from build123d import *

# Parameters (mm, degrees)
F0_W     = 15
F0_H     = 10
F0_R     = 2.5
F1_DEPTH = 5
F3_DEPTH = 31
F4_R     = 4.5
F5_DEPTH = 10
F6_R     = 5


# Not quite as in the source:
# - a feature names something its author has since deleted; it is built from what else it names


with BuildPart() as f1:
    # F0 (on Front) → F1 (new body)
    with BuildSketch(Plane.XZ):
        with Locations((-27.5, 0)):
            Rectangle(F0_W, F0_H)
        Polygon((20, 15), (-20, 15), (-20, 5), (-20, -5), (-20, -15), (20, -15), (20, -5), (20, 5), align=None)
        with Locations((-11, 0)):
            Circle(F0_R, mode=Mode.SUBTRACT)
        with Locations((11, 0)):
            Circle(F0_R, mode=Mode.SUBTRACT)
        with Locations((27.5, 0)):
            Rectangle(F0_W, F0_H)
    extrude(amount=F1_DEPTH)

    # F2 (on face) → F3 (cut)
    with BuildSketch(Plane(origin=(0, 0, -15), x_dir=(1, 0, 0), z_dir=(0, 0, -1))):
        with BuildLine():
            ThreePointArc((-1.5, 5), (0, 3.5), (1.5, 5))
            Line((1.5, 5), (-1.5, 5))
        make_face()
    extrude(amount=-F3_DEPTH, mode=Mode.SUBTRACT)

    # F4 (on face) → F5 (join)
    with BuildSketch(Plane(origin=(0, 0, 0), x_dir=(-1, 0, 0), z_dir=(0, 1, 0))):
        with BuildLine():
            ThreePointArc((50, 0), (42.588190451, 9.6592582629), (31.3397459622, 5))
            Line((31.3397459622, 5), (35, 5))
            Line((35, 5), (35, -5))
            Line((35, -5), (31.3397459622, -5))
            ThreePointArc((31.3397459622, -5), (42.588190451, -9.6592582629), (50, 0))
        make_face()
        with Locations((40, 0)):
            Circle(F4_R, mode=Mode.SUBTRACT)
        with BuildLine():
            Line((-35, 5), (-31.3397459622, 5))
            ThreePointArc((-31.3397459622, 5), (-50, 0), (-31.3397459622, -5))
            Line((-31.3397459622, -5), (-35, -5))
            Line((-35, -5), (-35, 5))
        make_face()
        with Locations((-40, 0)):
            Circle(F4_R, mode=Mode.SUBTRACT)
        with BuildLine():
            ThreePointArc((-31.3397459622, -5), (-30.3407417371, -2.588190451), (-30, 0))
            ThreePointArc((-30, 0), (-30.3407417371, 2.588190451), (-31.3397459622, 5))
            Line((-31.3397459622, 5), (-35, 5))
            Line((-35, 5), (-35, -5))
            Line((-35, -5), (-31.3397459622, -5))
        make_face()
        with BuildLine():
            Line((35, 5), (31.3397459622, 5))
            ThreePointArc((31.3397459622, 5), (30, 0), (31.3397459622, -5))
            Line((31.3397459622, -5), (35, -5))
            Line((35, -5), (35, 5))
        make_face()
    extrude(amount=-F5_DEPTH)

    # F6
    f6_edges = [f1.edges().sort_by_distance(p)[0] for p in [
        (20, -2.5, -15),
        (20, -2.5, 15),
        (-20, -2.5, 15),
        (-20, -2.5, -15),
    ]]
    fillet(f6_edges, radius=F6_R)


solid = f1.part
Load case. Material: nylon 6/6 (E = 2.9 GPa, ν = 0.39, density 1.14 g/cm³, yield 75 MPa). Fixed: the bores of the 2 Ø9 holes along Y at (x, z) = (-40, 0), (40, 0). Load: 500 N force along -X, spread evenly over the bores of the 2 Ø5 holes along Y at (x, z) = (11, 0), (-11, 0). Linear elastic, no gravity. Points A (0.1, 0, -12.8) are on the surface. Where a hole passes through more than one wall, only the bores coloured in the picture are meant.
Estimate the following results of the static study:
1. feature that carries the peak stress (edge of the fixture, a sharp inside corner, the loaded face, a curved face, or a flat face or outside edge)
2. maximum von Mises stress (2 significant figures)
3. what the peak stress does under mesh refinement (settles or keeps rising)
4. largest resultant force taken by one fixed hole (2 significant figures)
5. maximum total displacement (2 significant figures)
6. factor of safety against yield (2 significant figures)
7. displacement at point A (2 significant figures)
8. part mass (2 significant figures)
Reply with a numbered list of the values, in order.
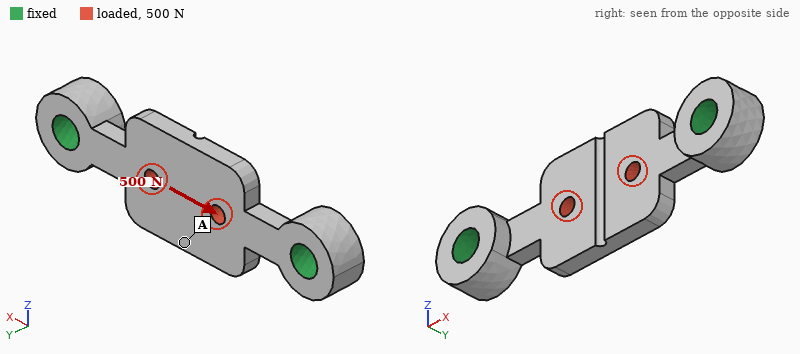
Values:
1. the loaded face
2. 7.7 MPa
3. settles
4. 250 N
5. 47 µm
6. 9.7
7. 33 µm
8. 13 g
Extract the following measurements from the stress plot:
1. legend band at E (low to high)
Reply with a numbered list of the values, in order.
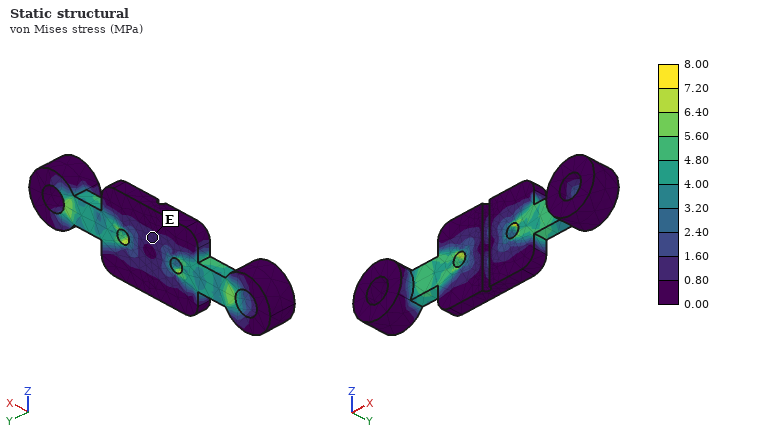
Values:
1. 0.80 to 1.60 MPa
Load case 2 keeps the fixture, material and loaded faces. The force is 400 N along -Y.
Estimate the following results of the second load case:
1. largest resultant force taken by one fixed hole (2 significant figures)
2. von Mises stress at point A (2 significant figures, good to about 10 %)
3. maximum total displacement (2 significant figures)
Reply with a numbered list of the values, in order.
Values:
1. 220 N
2. 25 MPa
3. 1.1 mm
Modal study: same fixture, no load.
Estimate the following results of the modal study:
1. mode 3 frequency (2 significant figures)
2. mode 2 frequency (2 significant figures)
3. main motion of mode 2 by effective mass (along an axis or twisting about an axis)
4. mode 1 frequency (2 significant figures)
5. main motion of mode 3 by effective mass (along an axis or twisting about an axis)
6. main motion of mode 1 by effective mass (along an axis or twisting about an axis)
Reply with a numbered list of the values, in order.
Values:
1. 3100 Hz
2. 1400 Hz
3. twisting about X
4. 1300 Hz
5. along Z
6. along Y
